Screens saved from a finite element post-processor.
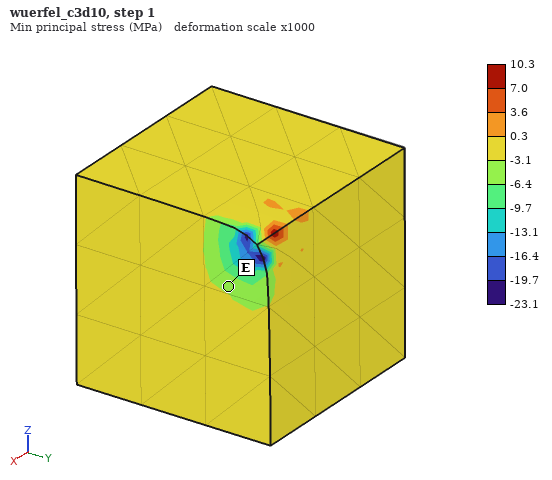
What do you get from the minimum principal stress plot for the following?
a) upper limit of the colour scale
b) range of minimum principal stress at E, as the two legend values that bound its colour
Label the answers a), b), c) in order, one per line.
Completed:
a) 10.3 MPa
b) -6.4 to -3.1 MPa
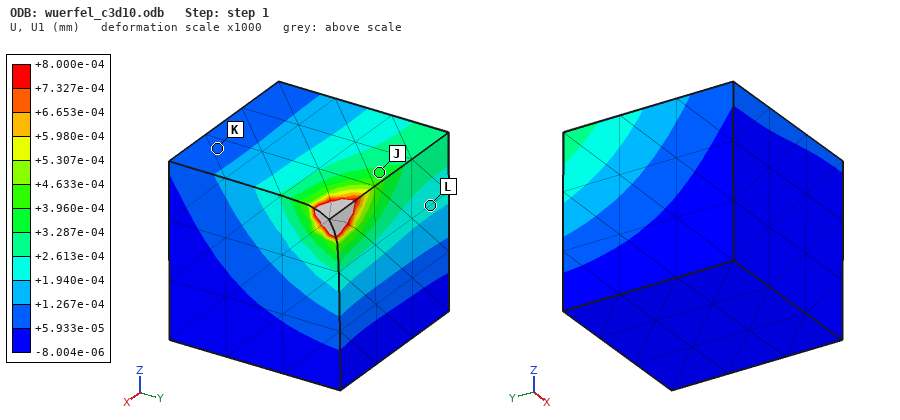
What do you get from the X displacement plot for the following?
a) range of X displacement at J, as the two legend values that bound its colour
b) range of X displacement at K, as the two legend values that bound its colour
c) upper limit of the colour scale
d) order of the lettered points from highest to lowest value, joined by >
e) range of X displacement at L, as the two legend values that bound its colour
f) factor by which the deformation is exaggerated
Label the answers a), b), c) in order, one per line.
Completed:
a) +3.287e-04 to +3.960e-04 mm
b) +5.933e-05 to +1.267e-04 mm
c) +8.000e-04 mm
d) J > L > K
e) +1.940e-04 to +2.613e-04 mm
f) 1000
